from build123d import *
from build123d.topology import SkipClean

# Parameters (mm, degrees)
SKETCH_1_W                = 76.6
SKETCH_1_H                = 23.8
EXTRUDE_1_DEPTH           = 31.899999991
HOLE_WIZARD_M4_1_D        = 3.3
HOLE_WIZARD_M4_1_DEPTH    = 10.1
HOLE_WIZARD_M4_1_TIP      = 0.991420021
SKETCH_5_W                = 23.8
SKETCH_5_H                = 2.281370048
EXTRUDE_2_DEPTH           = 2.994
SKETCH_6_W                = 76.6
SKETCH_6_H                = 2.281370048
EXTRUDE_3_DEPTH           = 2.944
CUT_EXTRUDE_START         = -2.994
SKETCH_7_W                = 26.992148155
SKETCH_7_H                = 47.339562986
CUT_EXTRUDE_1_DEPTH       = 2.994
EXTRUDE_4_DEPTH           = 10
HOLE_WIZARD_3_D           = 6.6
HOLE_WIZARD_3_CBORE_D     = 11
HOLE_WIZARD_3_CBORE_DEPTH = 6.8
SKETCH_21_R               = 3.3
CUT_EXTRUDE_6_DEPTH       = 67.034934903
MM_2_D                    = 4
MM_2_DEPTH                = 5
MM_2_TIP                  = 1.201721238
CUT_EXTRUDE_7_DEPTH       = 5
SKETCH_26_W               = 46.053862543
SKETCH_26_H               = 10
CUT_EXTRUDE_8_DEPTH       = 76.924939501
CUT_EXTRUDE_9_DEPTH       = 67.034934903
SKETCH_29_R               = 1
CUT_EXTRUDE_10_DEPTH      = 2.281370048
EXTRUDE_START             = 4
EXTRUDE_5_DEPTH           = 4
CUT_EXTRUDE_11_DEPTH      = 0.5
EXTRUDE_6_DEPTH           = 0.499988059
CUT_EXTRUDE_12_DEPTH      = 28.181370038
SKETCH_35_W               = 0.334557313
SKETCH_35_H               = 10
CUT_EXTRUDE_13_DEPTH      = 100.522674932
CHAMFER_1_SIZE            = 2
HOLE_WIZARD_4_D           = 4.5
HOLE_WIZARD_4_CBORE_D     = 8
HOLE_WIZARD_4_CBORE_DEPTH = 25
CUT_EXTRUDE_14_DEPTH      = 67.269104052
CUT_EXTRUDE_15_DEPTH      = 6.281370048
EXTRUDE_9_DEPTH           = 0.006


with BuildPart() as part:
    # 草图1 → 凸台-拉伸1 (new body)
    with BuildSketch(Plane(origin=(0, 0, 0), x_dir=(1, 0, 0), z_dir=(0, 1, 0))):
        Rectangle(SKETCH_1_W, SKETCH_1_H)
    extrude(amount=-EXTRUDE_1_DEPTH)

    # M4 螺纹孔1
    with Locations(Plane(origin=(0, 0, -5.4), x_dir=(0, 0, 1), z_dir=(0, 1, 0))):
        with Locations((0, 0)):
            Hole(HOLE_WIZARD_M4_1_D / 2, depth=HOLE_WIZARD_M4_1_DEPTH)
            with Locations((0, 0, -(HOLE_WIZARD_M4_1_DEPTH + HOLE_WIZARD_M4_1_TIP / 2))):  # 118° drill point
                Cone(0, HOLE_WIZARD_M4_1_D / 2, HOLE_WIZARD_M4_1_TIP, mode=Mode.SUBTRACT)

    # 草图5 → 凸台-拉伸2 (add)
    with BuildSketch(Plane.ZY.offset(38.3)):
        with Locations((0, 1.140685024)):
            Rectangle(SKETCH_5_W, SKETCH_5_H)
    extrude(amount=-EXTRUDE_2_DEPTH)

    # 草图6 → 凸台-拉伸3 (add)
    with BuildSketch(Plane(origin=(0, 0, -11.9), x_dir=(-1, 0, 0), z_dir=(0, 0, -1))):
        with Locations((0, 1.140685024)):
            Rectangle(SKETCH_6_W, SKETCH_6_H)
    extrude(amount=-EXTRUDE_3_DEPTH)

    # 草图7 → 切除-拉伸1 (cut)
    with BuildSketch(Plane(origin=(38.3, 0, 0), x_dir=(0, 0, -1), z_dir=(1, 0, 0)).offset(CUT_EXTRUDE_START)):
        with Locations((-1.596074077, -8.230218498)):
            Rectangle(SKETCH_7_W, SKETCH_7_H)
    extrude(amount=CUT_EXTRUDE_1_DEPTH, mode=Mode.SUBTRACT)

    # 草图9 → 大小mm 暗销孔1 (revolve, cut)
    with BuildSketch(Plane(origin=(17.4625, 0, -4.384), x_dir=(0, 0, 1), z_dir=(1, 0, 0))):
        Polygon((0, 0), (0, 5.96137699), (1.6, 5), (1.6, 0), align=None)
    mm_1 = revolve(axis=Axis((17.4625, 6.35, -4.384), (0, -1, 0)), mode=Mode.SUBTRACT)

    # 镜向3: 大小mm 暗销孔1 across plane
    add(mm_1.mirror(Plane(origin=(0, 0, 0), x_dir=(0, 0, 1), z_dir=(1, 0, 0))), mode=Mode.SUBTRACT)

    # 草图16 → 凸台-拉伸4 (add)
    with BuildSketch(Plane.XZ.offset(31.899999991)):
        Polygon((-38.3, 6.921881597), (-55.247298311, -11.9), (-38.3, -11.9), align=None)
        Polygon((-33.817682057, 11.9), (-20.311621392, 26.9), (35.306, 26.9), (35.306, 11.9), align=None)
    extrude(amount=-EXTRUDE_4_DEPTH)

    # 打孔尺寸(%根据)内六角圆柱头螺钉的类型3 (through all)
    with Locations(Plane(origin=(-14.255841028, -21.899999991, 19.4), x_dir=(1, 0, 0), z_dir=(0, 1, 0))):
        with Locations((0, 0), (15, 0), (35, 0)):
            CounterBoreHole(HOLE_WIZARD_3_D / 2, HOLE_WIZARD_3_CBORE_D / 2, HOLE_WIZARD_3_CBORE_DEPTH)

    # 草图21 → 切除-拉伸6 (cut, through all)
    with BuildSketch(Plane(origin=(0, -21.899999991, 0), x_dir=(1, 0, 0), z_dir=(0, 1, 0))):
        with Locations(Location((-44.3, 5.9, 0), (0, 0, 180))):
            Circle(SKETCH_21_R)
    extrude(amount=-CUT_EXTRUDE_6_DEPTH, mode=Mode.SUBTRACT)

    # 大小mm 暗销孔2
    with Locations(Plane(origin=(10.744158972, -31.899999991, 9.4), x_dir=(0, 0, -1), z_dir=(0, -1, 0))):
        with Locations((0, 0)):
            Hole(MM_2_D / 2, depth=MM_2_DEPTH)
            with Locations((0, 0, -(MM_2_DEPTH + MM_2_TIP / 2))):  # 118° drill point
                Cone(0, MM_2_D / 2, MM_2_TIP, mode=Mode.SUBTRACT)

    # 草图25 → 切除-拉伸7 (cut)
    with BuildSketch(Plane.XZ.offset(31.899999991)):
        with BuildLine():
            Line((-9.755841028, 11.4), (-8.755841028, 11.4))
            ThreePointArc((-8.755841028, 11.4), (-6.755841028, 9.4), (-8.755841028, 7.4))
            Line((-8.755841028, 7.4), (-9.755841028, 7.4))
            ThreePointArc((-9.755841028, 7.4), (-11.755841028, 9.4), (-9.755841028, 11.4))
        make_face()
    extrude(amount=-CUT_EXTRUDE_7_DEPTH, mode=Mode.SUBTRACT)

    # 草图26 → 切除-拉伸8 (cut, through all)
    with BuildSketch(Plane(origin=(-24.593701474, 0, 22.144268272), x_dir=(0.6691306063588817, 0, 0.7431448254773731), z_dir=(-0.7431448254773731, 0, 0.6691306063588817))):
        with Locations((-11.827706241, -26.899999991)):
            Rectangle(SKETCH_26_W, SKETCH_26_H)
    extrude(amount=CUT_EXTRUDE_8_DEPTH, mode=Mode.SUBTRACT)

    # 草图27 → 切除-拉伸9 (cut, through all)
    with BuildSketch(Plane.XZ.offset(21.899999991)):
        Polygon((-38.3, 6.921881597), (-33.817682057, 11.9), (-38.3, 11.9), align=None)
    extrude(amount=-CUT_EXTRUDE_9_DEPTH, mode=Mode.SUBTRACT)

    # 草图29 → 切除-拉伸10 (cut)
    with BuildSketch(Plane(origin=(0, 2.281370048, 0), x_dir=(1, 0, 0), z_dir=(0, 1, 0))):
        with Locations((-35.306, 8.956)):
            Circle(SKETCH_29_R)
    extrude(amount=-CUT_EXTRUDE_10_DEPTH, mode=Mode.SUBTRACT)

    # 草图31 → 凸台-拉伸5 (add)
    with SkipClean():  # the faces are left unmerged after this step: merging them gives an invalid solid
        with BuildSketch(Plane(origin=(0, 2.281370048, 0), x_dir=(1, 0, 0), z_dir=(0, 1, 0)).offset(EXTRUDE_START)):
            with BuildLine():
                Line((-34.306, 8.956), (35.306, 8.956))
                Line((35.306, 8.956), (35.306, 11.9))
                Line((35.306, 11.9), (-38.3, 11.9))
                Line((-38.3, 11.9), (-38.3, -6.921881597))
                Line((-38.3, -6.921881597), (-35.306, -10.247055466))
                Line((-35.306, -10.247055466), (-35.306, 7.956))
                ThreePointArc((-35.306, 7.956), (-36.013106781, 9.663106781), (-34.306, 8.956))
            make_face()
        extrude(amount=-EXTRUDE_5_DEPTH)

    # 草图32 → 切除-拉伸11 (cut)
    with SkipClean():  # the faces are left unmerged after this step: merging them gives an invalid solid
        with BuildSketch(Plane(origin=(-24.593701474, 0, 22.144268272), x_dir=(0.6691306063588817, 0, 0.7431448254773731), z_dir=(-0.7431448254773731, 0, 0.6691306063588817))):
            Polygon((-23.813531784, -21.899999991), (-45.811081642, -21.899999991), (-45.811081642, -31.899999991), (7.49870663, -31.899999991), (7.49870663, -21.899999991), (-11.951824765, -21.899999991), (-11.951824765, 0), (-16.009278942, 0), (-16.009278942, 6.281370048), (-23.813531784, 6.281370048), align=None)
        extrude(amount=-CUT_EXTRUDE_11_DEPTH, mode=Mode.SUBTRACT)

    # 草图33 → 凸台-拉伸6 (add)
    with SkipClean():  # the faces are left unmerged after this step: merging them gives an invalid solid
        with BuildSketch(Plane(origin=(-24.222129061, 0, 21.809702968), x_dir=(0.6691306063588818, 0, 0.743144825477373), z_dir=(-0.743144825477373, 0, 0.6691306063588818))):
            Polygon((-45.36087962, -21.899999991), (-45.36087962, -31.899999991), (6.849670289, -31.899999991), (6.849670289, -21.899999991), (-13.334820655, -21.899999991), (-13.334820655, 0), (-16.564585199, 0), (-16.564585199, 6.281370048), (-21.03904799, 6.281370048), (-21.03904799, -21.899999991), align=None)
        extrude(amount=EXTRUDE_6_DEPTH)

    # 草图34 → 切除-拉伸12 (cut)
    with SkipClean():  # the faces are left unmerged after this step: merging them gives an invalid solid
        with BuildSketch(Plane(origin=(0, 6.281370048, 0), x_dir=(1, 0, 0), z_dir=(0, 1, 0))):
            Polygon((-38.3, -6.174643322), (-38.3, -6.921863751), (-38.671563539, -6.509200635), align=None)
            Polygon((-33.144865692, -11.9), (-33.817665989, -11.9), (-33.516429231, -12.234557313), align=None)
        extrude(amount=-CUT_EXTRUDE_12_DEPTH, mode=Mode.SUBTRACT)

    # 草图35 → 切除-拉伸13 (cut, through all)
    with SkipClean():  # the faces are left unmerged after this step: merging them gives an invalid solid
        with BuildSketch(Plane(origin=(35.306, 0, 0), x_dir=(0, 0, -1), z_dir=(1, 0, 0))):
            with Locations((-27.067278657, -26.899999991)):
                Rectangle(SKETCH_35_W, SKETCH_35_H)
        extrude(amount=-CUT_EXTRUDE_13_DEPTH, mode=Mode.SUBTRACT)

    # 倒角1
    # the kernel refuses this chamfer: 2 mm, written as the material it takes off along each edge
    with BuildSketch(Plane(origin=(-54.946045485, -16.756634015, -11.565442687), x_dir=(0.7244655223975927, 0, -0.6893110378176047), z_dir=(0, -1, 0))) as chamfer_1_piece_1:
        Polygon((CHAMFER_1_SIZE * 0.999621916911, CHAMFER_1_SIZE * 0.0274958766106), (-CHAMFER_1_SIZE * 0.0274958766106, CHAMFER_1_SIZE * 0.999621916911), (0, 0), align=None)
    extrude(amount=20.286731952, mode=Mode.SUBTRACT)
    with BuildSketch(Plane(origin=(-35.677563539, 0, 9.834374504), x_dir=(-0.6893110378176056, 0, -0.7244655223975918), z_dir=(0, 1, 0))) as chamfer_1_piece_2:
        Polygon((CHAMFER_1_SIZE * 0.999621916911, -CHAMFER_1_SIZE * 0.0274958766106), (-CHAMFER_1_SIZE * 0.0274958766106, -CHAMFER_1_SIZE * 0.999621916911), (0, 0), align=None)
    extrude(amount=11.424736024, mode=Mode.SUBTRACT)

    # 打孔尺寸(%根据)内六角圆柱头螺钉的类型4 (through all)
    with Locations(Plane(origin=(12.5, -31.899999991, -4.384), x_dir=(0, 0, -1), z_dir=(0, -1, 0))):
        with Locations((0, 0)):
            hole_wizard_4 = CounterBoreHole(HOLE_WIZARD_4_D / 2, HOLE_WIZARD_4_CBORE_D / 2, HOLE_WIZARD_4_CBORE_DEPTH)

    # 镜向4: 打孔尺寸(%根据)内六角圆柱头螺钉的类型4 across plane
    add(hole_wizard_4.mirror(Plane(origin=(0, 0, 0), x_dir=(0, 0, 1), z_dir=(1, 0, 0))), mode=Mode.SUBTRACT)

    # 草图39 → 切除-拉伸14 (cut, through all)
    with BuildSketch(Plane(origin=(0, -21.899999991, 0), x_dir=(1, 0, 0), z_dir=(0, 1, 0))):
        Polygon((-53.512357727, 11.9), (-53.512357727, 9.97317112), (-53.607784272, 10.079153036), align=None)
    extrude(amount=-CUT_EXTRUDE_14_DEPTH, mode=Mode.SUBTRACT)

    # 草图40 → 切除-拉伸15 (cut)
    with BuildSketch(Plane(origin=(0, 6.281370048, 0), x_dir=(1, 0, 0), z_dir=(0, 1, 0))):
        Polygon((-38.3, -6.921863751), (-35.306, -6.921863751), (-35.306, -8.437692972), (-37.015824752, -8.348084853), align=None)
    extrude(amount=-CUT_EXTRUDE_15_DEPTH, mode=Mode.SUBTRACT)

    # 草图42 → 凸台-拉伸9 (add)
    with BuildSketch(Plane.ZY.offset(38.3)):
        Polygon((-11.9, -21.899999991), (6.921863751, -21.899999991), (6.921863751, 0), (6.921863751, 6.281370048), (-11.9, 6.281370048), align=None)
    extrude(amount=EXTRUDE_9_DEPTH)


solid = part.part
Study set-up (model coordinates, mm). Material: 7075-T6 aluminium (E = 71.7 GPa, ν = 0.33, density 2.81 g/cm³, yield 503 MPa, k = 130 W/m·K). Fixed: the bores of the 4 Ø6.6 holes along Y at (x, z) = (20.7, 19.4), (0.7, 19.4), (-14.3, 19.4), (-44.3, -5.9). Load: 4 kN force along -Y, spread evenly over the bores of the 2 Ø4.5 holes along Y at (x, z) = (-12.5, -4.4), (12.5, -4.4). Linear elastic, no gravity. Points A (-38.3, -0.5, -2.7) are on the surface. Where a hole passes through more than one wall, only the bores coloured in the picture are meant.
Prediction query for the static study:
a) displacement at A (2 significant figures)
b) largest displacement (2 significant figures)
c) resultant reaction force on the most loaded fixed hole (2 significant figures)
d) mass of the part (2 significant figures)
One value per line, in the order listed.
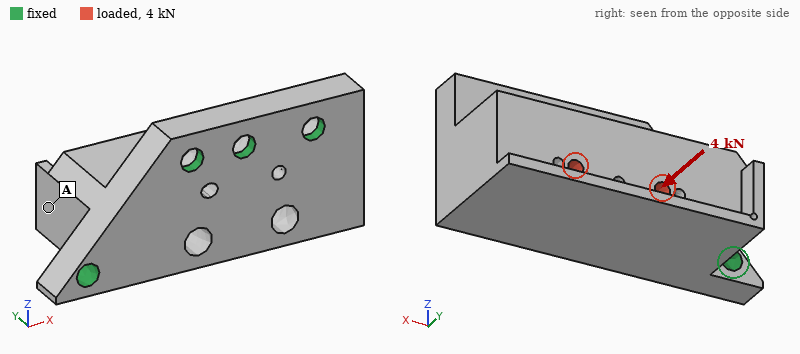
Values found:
0.049 mm
0.13 mm
2.7 kN
180 g
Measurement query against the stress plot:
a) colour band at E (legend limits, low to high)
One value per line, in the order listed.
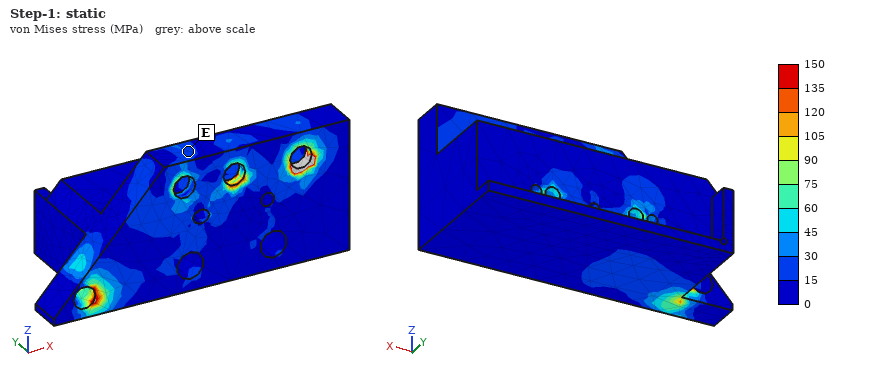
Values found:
15 to 30 MPa
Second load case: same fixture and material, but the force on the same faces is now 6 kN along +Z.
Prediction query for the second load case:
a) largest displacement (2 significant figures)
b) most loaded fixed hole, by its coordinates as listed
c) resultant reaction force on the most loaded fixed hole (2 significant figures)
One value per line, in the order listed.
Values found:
0.26 mm
(-14.3, 19.4)
5.3 kN
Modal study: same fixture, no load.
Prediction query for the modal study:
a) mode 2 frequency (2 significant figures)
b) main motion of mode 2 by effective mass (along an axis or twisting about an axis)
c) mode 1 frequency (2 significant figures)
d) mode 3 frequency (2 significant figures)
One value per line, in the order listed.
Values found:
9900 Hz
along X
3000 Hz
10 kHz
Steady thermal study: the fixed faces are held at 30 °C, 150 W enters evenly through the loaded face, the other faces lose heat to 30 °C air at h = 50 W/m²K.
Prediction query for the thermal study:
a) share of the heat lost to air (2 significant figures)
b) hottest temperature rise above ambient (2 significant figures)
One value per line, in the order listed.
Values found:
13 %
62 K
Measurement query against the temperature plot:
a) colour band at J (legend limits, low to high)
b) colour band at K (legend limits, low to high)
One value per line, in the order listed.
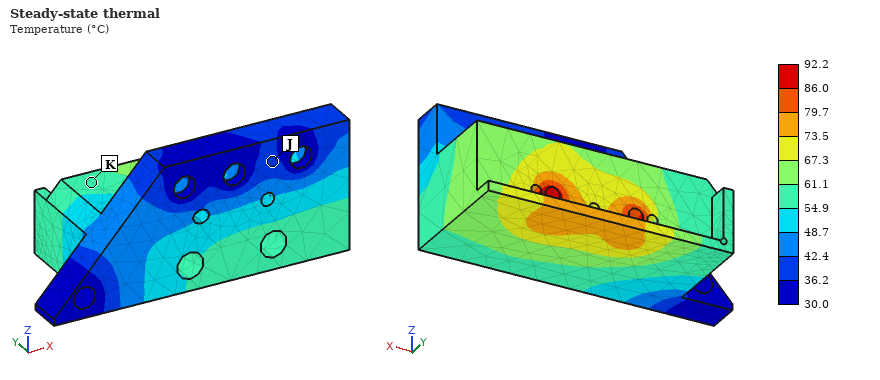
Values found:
36.2 to 42.4 °C
54.9 to 61.1 °C
